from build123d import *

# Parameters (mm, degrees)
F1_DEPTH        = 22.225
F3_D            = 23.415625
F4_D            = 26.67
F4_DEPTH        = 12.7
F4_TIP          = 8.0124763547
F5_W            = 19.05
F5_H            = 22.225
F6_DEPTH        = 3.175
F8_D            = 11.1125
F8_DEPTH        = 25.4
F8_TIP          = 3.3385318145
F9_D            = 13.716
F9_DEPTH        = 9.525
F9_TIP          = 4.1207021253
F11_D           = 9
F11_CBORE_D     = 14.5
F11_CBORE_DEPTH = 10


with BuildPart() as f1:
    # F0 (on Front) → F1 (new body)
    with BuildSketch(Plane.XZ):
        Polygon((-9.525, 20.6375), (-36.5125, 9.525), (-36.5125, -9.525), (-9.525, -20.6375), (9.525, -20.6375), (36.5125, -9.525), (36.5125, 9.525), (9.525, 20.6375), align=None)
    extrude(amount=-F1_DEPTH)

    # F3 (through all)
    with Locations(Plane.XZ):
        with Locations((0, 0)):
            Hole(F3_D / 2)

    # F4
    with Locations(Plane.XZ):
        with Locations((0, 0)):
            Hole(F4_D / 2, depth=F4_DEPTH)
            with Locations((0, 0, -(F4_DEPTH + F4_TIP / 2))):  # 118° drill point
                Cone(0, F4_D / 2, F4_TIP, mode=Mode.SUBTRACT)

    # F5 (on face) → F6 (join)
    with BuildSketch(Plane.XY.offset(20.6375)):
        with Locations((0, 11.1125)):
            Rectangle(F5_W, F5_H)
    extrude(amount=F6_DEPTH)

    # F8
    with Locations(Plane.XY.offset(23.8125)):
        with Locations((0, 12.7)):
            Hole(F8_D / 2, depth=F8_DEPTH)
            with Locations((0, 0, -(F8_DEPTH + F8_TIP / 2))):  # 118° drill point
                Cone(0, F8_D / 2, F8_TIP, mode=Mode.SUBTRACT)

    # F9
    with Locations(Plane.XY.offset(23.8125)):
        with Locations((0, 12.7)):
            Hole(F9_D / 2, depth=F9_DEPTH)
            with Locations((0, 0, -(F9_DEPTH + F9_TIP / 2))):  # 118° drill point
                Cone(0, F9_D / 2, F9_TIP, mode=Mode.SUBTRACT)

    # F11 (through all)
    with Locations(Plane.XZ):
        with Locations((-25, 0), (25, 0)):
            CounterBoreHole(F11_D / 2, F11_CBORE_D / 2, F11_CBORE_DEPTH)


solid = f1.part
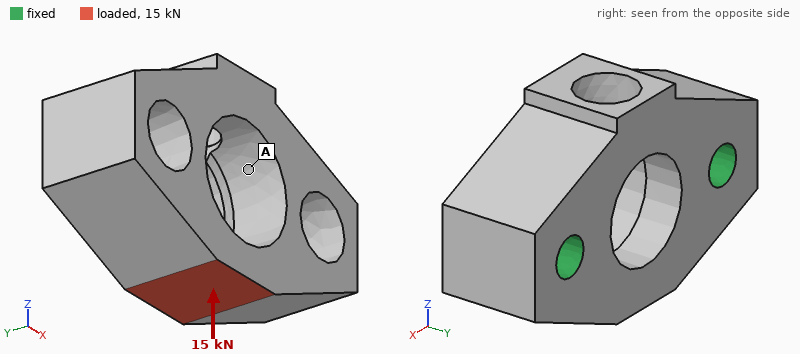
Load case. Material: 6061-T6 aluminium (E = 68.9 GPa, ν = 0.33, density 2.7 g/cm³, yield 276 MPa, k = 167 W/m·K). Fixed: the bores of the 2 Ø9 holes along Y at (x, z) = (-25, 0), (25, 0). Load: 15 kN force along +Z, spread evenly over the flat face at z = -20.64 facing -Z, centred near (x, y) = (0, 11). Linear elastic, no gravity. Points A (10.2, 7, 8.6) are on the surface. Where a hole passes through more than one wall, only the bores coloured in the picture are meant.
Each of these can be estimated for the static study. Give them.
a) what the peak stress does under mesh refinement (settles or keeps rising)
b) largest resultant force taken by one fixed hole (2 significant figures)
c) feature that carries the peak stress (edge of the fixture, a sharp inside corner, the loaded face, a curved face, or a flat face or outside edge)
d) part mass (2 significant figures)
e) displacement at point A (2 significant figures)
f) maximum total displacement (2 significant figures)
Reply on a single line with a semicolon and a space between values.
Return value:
keeps rising; 9.0 kN; edge of the fixture; 100 g; 9.8 µm; 63 µm
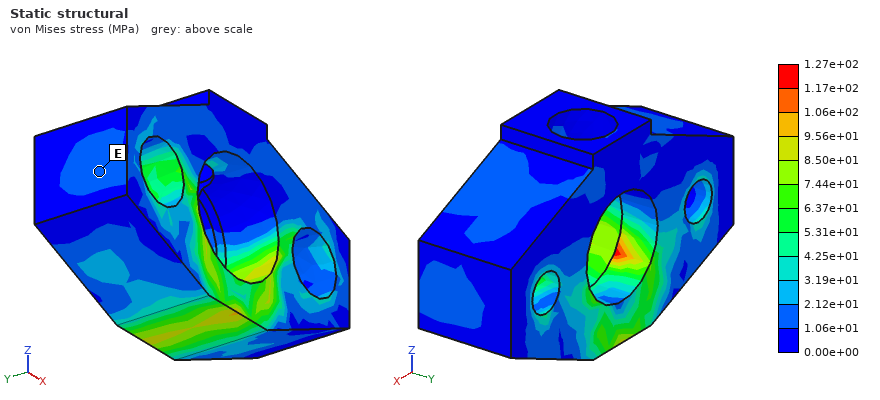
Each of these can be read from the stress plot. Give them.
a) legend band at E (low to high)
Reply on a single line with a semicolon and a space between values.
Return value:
1.06e+01 to 2.12e+01 MPa
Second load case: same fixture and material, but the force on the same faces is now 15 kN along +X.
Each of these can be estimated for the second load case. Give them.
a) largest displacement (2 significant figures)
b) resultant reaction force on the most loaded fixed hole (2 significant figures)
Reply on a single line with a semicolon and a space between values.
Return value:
24 µm; 9.0 kN
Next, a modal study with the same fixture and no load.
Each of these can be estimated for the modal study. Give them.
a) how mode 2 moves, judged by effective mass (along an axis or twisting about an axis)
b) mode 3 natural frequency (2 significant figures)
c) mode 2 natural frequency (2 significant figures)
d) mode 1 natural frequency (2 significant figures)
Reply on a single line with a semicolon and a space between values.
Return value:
along Y; 22 kHz; 17 kHz; 13 kHz
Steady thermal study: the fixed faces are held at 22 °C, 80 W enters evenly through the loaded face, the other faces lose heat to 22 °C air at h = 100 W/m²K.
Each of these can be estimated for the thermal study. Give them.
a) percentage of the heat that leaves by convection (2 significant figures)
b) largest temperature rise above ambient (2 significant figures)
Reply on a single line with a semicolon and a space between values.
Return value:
6.2 %; 26 K
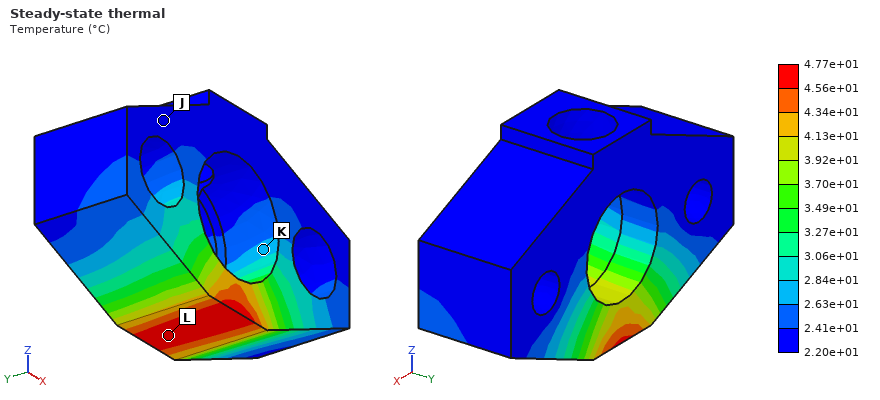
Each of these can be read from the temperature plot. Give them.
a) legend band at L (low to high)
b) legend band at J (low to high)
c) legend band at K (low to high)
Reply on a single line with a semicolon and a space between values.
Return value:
4.56e+01 to 4.77e+01 °C; 2.20e+01 to 2.41e+01 °C; 2.63e+01 to 2.84e+01 °C
